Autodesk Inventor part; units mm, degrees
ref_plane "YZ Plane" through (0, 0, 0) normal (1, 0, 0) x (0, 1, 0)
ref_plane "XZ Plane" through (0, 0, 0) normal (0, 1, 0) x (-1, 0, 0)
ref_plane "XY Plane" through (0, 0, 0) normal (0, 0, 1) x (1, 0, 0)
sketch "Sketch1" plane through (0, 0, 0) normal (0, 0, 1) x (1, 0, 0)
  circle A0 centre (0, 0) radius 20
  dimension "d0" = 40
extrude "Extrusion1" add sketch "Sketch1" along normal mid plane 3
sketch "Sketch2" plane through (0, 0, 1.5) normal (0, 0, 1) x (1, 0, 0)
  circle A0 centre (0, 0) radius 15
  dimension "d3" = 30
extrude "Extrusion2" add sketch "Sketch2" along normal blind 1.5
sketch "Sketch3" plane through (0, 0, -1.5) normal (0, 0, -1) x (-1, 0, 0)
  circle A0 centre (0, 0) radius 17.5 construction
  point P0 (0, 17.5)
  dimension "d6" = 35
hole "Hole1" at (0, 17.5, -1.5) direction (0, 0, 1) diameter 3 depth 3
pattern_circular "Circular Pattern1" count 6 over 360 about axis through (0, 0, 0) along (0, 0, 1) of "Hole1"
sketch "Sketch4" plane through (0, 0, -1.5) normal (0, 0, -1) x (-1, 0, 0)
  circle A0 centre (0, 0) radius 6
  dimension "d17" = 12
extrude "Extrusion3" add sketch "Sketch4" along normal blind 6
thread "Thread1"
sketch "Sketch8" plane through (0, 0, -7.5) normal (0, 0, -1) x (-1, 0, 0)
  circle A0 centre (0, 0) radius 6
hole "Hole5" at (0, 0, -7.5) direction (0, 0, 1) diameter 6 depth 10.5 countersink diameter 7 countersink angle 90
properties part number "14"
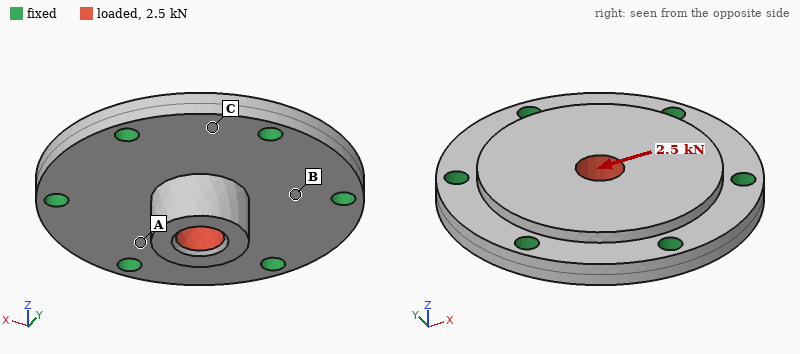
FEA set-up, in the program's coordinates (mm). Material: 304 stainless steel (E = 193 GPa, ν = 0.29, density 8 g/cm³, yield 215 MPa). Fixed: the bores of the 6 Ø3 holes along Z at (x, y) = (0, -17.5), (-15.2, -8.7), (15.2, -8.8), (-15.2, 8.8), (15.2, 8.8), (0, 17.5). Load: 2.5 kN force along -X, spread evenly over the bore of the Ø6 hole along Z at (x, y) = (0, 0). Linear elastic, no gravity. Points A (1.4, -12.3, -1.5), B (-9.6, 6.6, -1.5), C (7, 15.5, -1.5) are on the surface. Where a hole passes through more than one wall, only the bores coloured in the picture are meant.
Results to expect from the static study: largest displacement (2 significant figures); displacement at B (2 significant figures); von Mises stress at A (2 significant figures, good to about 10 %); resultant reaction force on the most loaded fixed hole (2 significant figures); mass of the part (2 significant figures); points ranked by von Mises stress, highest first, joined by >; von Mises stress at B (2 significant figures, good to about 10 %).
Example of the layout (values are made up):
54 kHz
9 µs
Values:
5.4 µm
0.95 µm
14 MPa
540 N
41 g
B > A > C
28 MPa
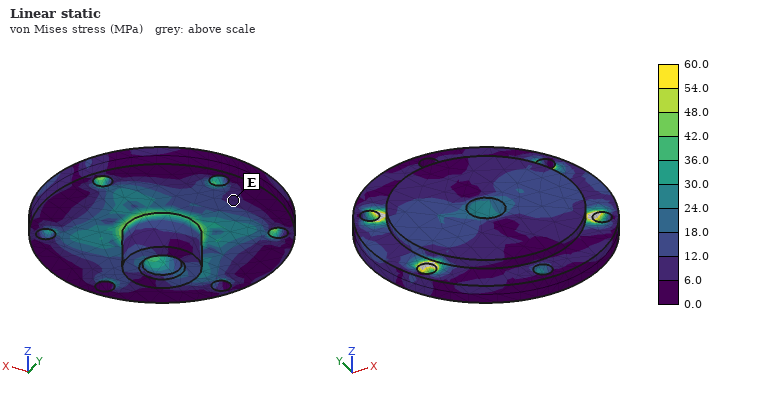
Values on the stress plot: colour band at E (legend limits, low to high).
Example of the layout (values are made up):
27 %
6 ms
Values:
6.0 to 12.0 MPa
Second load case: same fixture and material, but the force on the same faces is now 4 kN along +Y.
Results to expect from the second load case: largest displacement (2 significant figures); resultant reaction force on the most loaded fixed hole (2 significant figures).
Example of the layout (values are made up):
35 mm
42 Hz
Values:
8.6 µm
970 N
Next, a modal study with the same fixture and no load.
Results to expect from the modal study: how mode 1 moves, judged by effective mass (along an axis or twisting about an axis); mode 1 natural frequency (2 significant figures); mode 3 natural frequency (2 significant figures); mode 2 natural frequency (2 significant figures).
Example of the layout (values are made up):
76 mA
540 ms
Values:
along Z
21 kHz
35 kHz
35 kHz
